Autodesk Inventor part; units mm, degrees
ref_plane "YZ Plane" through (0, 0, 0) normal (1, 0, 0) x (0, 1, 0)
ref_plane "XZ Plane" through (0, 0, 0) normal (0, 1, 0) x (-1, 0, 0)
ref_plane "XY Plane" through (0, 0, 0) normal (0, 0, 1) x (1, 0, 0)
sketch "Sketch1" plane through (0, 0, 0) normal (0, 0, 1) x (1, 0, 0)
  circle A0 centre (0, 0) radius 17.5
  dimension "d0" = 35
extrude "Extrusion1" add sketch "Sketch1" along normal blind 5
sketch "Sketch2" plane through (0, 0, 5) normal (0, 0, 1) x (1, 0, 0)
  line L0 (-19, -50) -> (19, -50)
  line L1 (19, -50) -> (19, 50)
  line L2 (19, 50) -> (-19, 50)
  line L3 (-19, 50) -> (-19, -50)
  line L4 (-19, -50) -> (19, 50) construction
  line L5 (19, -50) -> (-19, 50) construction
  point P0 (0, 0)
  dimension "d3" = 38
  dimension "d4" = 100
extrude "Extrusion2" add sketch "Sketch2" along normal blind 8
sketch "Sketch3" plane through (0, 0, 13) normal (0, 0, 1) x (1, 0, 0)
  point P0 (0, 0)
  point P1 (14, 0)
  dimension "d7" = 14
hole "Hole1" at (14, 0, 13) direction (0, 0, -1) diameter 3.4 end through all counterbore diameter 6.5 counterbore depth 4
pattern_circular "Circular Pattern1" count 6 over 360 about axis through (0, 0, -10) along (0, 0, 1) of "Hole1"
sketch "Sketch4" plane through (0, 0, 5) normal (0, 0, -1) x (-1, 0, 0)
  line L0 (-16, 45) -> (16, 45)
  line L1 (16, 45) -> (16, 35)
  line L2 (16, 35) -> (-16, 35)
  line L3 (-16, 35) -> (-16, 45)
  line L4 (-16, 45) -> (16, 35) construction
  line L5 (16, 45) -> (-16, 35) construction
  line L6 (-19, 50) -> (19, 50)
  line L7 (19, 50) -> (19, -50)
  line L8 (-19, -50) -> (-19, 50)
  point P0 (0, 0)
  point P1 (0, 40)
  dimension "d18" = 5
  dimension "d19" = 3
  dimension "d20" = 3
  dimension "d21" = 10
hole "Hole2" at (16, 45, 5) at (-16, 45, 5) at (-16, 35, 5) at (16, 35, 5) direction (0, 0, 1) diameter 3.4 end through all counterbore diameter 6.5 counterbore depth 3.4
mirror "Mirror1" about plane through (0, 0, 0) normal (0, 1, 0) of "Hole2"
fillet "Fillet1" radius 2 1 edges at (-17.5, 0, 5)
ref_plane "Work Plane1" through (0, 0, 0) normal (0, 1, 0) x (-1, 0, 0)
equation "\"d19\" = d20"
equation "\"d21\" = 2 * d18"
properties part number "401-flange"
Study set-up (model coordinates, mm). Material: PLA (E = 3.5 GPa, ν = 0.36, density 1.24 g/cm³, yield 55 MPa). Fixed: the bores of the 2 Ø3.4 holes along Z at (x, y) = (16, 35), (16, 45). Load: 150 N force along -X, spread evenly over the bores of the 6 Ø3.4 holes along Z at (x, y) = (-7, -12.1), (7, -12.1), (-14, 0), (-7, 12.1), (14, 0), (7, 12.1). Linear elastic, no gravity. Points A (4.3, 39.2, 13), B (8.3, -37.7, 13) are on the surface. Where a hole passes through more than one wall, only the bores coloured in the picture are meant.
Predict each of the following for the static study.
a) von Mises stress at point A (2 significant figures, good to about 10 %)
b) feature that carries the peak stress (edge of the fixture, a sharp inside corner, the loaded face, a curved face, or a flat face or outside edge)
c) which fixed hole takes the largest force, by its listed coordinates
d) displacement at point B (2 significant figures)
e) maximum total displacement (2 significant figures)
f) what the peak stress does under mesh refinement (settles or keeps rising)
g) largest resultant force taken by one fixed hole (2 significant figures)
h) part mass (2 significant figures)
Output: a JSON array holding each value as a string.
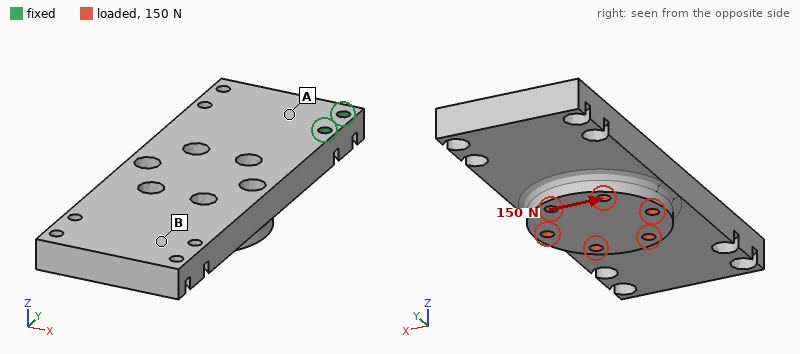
["6.4 MPa", "edge of the fixture", "(16, 35)", "0.51 mm", "0.76 mm", "keeps rising", "540 N", "41 g"]
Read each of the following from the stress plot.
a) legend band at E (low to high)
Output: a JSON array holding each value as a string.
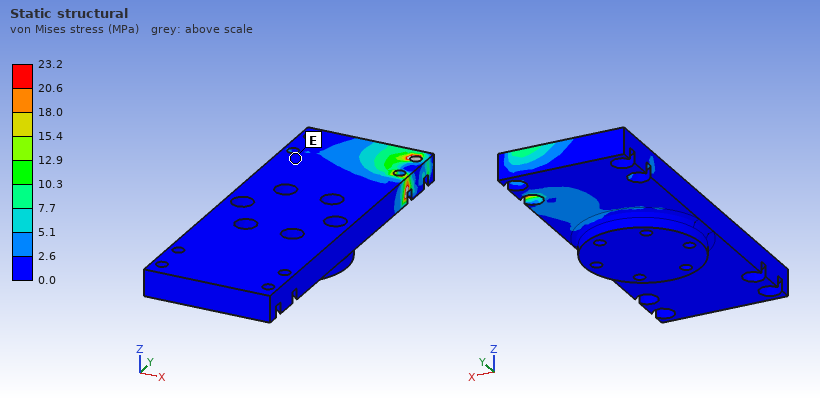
["0.0 to 2.6 MPa"]
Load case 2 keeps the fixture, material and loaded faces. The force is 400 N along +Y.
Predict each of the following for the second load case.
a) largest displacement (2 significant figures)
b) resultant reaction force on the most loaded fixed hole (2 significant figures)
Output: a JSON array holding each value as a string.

["1.2 mm", "560 N"]
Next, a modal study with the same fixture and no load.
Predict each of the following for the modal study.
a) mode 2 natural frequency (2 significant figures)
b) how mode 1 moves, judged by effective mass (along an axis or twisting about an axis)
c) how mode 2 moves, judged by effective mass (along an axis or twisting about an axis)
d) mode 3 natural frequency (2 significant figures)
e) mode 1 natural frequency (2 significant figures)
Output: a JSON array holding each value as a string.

["480 Hz", "along Z", "along X", "710 Hz", "210 Hz"]
